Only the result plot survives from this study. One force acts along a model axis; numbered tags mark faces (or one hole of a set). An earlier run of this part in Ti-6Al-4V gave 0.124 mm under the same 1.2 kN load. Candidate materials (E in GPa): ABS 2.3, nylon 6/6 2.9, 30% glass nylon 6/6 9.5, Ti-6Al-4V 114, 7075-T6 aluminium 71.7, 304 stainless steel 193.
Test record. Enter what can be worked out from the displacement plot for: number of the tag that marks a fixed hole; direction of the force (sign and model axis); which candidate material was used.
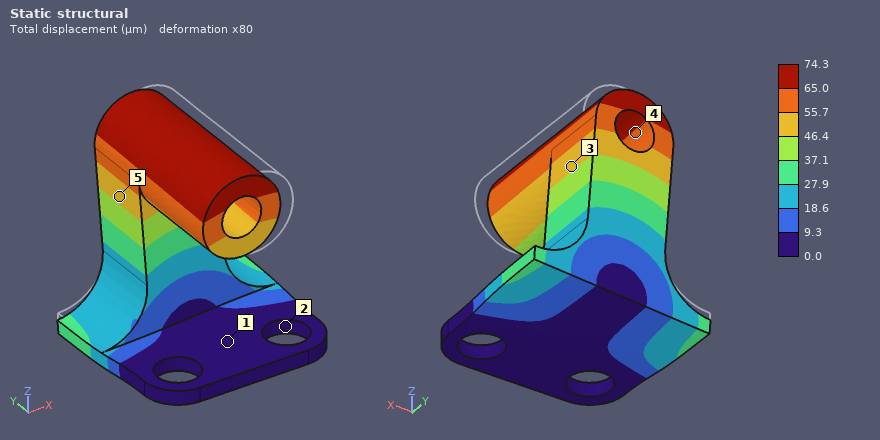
2
-X
304 stainless steel
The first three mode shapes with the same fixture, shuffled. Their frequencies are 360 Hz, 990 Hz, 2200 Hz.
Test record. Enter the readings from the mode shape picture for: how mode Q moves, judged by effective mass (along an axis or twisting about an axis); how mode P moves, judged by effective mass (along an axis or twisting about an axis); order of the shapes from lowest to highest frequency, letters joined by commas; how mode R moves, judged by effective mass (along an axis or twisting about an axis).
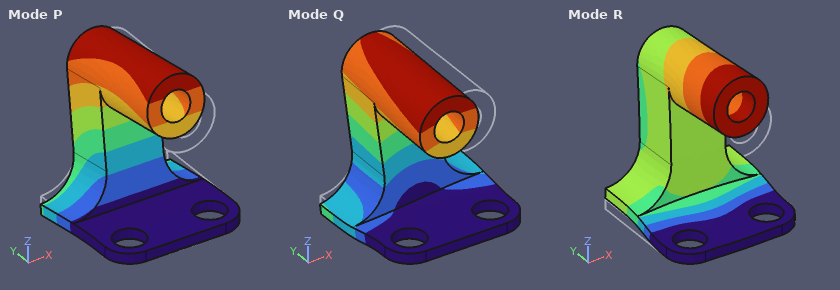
along X
along Y
P, Q, R
along Z
